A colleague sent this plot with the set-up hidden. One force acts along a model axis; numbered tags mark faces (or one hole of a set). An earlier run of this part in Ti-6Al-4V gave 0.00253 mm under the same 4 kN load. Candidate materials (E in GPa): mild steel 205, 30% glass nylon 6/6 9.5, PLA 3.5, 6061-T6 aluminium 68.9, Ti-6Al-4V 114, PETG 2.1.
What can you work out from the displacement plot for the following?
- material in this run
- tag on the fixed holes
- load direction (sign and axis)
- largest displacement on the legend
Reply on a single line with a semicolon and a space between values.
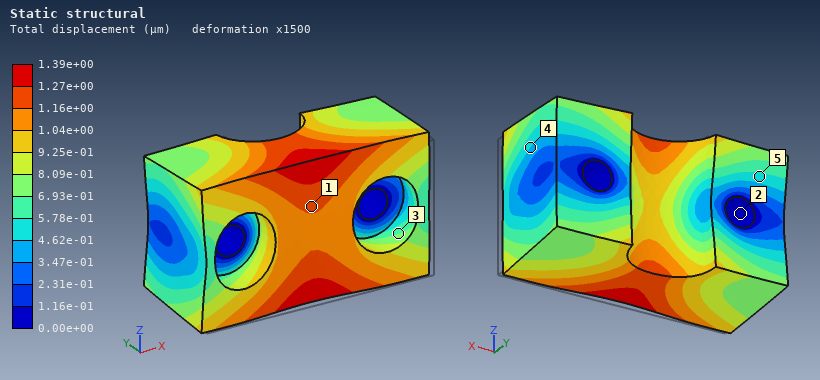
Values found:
mild steel; 2; +Y; 1.39e+00 µm
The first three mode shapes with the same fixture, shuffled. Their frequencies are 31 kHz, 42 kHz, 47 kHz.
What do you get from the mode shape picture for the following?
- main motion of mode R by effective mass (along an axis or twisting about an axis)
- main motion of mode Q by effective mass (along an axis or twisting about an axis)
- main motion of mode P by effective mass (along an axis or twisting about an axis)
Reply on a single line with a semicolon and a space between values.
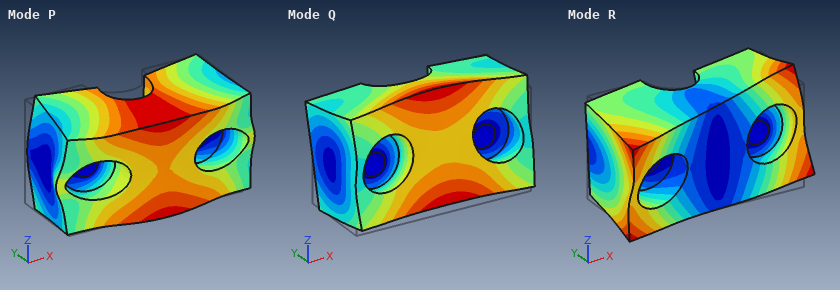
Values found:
twisting about Y; along Z; along Y
